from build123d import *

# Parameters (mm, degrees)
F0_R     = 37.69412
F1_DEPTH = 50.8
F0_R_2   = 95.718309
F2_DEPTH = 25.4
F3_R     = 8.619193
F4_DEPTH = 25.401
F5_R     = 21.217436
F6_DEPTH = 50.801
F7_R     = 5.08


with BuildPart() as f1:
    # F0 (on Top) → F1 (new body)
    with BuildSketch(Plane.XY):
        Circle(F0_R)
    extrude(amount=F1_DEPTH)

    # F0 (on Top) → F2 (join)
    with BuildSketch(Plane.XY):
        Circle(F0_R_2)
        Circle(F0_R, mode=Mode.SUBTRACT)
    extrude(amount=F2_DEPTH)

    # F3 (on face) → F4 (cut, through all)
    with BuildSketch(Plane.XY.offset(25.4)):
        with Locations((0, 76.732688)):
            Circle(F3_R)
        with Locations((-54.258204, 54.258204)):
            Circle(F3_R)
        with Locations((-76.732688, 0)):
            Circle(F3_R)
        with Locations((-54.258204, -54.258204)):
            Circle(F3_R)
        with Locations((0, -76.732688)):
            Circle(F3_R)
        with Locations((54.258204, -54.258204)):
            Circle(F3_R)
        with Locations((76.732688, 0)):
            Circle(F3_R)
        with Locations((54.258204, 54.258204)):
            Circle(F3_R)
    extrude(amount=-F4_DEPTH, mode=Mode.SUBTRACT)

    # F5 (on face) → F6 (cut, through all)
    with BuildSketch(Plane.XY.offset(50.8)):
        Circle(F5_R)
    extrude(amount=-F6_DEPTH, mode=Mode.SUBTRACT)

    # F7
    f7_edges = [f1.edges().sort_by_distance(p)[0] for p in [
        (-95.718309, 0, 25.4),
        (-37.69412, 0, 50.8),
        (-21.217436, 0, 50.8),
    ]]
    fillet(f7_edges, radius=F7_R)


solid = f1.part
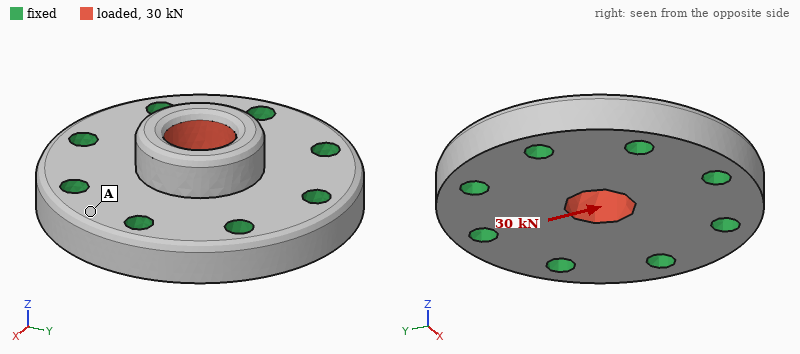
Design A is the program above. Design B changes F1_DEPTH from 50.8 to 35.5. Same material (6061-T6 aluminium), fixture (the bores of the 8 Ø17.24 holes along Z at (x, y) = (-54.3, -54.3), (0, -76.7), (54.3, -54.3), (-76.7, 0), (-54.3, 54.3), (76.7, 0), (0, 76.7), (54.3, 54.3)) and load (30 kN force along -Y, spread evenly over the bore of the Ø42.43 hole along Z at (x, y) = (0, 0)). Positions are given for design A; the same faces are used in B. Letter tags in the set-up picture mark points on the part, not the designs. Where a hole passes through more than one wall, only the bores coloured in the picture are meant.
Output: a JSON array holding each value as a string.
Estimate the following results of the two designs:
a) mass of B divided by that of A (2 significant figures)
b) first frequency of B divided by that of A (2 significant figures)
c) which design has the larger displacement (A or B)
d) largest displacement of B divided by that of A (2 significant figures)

["0.94", "1.1", "A", "0.53"]
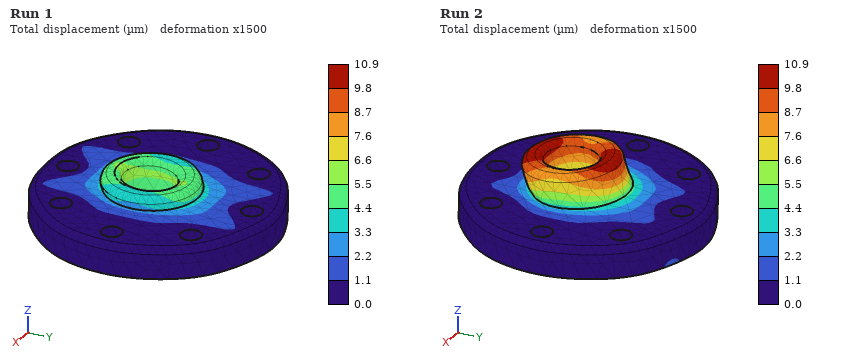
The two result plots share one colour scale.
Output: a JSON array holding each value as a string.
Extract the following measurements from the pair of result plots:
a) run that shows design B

["Run 1"]
